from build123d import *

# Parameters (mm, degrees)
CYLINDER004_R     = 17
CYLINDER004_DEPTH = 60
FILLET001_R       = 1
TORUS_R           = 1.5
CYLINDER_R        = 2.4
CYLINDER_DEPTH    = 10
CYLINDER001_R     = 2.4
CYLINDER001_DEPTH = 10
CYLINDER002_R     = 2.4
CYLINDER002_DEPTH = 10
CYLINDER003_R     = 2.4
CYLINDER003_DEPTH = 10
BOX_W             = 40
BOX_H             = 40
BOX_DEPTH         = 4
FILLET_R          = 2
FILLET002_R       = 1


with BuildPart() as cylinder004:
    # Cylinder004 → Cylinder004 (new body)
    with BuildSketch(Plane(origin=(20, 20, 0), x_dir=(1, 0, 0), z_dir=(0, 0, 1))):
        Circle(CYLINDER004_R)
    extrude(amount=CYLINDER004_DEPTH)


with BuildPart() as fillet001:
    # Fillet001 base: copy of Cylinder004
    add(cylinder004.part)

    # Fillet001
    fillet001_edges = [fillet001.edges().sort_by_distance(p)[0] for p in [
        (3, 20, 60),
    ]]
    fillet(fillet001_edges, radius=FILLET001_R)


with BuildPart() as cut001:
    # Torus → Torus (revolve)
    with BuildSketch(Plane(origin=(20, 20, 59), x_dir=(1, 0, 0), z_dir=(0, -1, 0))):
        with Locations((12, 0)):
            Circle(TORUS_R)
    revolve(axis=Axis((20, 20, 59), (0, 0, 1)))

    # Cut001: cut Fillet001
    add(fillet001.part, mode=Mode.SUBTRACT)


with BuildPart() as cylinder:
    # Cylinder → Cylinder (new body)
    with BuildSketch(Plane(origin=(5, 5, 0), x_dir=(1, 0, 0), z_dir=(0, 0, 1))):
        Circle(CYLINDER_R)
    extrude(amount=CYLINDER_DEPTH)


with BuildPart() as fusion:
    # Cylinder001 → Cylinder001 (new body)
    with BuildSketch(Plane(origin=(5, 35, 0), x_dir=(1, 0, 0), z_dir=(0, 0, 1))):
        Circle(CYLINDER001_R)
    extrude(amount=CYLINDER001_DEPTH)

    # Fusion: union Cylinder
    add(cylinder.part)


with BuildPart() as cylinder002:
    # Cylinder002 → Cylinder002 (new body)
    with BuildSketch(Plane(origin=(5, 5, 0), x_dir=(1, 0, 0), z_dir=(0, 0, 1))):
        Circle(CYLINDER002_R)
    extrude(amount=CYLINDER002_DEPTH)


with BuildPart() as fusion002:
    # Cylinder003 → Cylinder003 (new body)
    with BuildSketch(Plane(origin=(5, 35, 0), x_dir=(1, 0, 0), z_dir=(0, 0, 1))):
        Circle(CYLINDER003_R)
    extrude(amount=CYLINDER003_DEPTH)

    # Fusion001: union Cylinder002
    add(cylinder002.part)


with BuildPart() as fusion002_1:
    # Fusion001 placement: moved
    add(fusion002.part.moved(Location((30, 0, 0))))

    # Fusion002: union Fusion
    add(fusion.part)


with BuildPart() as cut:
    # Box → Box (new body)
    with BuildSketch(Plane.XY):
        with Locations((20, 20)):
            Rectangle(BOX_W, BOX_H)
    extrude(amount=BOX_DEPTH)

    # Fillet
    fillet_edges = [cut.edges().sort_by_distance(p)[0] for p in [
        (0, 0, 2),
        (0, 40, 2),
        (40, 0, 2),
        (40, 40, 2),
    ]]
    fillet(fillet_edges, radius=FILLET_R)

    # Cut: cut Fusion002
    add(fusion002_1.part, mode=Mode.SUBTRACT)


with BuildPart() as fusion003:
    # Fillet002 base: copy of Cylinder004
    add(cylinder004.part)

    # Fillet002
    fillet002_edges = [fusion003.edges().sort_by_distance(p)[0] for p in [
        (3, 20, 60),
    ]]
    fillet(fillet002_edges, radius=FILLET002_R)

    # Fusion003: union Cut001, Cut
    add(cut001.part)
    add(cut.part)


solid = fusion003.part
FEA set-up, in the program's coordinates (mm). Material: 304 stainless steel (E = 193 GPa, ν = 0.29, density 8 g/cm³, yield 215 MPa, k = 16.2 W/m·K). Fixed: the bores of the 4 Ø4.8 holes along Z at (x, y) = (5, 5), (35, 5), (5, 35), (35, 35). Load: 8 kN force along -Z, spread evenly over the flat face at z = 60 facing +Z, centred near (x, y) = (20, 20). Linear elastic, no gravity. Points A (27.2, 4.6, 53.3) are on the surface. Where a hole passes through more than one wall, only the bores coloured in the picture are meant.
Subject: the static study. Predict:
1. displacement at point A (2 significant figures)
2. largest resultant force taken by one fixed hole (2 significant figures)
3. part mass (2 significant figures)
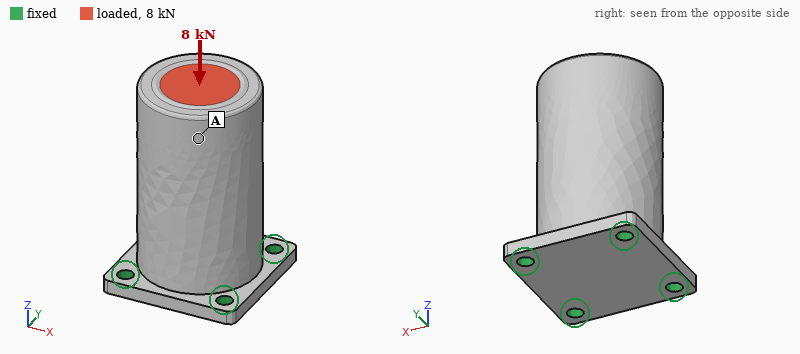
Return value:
6.8 µm
2.2 kN
460 g
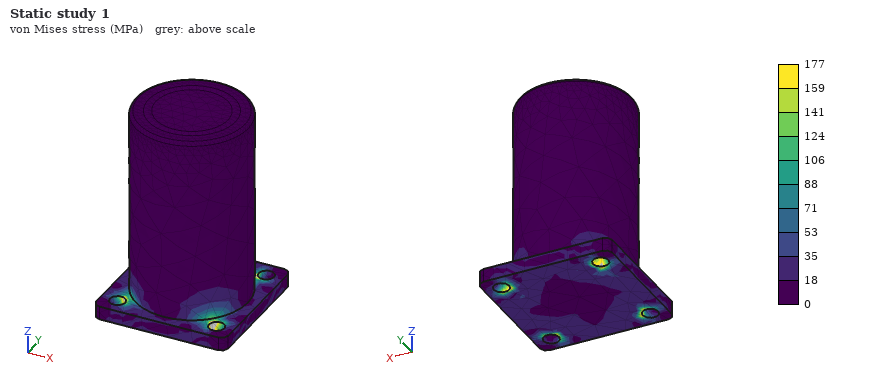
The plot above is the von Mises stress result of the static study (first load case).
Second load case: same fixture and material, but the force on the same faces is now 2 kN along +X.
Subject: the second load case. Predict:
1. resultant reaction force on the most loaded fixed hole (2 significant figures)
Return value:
2.3 kN
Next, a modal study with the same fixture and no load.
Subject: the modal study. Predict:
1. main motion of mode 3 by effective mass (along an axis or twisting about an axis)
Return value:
along Z
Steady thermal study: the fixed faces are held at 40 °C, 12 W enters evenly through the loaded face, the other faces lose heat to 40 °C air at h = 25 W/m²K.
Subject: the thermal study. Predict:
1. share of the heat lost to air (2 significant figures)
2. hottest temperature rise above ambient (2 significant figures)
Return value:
42 %
53 K
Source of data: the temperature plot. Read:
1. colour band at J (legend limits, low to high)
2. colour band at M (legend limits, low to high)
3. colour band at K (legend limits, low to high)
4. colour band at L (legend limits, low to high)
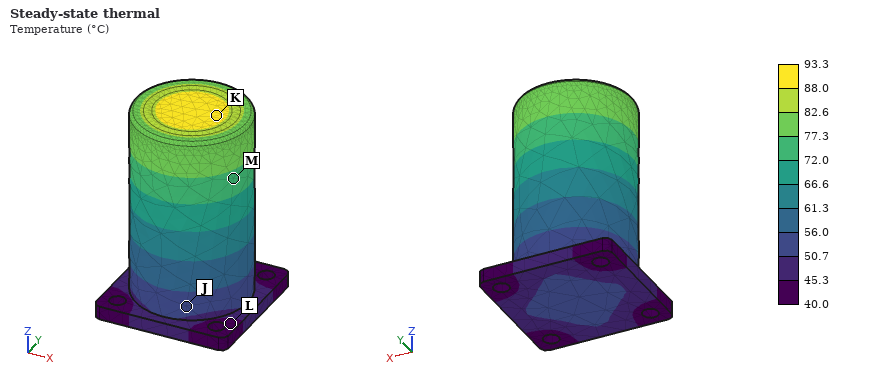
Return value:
50.7 to 56.0 °C
72.0 to 77.3 °C
88.0 to 93.3 °C
40.0 to 45.3 °C
